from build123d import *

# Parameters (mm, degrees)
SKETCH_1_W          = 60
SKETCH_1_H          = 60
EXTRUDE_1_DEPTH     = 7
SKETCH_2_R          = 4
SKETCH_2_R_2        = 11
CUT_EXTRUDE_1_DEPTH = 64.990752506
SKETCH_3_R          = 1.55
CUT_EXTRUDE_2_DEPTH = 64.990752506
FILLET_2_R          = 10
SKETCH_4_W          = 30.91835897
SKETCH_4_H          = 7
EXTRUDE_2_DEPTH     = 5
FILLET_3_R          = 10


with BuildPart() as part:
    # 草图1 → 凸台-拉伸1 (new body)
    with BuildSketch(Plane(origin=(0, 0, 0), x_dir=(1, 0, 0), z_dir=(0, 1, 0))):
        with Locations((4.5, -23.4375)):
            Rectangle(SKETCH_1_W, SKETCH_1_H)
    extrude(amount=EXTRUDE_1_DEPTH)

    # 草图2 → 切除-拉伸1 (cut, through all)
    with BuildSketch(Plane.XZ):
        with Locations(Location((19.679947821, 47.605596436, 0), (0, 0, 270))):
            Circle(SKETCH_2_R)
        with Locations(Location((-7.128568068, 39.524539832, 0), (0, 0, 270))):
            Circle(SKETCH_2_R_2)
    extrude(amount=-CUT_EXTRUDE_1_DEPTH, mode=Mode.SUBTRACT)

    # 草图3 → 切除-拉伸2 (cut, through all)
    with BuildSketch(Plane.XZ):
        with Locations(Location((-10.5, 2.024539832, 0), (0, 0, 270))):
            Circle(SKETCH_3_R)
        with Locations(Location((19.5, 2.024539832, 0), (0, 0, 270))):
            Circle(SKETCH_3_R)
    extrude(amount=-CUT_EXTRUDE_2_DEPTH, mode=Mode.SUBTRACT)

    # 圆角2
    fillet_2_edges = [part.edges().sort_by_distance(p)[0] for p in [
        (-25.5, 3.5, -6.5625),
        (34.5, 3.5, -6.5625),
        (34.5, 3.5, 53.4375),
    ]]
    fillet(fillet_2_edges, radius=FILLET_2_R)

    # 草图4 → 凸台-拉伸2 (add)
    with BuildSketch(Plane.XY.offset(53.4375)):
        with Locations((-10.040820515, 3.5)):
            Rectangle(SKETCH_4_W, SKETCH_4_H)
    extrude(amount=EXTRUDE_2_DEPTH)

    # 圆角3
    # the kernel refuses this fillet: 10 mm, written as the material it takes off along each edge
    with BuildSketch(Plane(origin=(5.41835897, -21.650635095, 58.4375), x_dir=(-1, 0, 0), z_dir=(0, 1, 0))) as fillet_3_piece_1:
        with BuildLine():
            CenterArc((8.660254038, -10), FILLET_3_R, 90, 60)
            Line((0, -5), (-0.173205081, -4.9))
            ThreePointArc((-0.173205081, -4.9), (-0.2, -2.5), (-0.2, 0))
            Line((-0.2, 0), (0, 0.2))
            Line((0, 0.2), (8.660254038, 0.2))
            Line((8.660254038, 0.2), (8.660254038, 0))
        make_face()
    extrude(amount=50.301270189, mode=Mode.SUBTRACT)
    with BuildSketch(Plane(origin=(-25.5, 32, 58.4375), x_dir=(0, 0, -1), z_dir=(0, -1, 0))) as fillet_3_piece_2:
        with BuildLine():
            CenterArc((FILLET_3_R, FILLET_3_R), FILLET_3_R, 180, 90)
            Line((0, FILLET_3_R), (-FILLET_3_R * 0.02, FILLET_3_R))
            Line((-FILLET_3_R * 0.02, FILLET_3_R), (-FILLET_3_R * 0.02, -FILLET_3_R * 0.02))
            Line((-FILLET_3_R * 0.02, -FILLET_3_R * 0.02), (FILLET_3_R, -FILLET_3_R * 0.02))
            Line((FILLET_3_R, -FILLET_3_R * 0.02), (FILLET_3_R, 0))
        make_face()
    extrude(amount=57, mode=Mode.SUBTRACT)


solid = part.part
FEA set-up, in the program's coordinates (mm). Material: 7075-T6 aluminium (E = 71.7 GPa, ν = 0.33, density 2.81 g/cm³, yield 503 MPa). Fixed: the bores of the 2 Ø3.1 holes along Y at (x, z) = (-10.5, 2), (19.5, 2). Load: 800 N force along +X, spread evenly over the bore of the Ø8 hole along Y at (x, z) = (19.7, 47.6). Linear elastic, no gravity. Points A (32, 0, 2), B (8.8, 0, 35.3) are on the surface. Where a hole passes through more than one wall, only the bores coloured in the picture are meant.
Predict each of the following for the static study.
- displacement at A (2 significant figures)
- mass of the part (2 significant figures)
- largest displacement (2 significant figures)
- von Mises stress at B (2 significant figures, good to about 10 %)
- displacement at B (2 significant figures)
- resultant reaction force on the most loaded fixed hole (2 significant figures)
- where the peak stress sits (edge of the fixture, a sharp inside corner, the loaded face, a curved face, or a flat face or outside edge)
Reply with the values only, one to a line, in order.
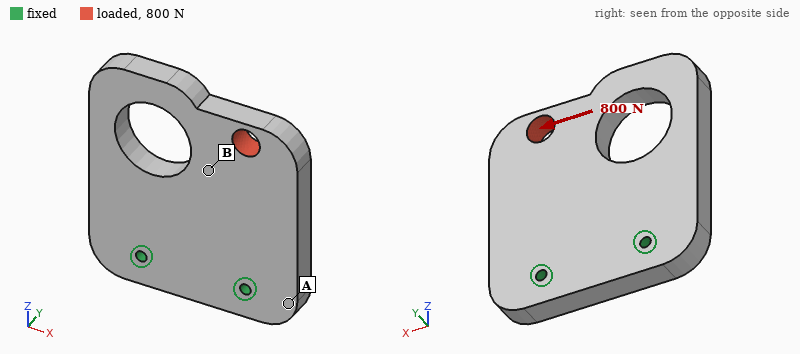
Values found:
4.4 µm
63 g
19 µm
8.8 MPa
9.4 µm
1.2 kN
edge of the fixture
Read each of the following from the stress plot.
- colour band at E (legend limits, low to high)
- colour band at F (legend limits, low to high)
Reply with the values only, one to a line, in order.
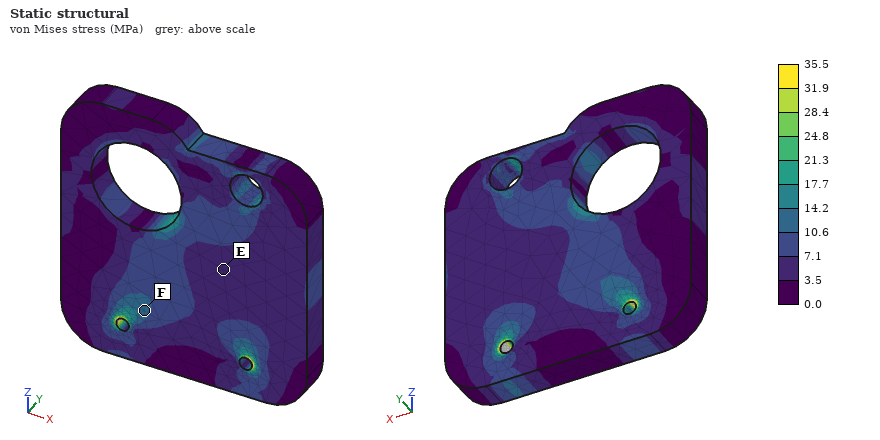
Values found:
3.5 to 7.1 MPa
10.6 to 14.2 MPa
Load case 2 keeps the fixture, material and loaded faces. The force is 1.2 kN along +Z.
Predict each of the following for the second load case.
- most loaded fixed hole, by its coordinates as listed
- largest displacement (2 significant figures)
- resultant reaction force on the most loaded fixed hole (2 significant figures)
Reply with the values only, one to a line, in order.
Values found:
(19.5, 2)
9.6 µm
1.2 kN
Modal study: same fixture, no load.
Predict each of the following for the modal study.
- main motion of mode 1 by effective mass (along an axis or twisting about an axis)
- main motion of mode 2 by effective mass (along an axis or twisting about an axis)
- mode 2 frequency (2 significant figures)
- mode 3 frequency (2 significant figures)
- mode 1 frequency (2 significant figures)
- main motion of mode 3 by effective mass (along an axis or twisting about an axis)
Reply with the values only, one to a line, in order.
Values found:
along Y
twisting about Z
3900 Hz
7600 Hz
1900 Hz
along X
